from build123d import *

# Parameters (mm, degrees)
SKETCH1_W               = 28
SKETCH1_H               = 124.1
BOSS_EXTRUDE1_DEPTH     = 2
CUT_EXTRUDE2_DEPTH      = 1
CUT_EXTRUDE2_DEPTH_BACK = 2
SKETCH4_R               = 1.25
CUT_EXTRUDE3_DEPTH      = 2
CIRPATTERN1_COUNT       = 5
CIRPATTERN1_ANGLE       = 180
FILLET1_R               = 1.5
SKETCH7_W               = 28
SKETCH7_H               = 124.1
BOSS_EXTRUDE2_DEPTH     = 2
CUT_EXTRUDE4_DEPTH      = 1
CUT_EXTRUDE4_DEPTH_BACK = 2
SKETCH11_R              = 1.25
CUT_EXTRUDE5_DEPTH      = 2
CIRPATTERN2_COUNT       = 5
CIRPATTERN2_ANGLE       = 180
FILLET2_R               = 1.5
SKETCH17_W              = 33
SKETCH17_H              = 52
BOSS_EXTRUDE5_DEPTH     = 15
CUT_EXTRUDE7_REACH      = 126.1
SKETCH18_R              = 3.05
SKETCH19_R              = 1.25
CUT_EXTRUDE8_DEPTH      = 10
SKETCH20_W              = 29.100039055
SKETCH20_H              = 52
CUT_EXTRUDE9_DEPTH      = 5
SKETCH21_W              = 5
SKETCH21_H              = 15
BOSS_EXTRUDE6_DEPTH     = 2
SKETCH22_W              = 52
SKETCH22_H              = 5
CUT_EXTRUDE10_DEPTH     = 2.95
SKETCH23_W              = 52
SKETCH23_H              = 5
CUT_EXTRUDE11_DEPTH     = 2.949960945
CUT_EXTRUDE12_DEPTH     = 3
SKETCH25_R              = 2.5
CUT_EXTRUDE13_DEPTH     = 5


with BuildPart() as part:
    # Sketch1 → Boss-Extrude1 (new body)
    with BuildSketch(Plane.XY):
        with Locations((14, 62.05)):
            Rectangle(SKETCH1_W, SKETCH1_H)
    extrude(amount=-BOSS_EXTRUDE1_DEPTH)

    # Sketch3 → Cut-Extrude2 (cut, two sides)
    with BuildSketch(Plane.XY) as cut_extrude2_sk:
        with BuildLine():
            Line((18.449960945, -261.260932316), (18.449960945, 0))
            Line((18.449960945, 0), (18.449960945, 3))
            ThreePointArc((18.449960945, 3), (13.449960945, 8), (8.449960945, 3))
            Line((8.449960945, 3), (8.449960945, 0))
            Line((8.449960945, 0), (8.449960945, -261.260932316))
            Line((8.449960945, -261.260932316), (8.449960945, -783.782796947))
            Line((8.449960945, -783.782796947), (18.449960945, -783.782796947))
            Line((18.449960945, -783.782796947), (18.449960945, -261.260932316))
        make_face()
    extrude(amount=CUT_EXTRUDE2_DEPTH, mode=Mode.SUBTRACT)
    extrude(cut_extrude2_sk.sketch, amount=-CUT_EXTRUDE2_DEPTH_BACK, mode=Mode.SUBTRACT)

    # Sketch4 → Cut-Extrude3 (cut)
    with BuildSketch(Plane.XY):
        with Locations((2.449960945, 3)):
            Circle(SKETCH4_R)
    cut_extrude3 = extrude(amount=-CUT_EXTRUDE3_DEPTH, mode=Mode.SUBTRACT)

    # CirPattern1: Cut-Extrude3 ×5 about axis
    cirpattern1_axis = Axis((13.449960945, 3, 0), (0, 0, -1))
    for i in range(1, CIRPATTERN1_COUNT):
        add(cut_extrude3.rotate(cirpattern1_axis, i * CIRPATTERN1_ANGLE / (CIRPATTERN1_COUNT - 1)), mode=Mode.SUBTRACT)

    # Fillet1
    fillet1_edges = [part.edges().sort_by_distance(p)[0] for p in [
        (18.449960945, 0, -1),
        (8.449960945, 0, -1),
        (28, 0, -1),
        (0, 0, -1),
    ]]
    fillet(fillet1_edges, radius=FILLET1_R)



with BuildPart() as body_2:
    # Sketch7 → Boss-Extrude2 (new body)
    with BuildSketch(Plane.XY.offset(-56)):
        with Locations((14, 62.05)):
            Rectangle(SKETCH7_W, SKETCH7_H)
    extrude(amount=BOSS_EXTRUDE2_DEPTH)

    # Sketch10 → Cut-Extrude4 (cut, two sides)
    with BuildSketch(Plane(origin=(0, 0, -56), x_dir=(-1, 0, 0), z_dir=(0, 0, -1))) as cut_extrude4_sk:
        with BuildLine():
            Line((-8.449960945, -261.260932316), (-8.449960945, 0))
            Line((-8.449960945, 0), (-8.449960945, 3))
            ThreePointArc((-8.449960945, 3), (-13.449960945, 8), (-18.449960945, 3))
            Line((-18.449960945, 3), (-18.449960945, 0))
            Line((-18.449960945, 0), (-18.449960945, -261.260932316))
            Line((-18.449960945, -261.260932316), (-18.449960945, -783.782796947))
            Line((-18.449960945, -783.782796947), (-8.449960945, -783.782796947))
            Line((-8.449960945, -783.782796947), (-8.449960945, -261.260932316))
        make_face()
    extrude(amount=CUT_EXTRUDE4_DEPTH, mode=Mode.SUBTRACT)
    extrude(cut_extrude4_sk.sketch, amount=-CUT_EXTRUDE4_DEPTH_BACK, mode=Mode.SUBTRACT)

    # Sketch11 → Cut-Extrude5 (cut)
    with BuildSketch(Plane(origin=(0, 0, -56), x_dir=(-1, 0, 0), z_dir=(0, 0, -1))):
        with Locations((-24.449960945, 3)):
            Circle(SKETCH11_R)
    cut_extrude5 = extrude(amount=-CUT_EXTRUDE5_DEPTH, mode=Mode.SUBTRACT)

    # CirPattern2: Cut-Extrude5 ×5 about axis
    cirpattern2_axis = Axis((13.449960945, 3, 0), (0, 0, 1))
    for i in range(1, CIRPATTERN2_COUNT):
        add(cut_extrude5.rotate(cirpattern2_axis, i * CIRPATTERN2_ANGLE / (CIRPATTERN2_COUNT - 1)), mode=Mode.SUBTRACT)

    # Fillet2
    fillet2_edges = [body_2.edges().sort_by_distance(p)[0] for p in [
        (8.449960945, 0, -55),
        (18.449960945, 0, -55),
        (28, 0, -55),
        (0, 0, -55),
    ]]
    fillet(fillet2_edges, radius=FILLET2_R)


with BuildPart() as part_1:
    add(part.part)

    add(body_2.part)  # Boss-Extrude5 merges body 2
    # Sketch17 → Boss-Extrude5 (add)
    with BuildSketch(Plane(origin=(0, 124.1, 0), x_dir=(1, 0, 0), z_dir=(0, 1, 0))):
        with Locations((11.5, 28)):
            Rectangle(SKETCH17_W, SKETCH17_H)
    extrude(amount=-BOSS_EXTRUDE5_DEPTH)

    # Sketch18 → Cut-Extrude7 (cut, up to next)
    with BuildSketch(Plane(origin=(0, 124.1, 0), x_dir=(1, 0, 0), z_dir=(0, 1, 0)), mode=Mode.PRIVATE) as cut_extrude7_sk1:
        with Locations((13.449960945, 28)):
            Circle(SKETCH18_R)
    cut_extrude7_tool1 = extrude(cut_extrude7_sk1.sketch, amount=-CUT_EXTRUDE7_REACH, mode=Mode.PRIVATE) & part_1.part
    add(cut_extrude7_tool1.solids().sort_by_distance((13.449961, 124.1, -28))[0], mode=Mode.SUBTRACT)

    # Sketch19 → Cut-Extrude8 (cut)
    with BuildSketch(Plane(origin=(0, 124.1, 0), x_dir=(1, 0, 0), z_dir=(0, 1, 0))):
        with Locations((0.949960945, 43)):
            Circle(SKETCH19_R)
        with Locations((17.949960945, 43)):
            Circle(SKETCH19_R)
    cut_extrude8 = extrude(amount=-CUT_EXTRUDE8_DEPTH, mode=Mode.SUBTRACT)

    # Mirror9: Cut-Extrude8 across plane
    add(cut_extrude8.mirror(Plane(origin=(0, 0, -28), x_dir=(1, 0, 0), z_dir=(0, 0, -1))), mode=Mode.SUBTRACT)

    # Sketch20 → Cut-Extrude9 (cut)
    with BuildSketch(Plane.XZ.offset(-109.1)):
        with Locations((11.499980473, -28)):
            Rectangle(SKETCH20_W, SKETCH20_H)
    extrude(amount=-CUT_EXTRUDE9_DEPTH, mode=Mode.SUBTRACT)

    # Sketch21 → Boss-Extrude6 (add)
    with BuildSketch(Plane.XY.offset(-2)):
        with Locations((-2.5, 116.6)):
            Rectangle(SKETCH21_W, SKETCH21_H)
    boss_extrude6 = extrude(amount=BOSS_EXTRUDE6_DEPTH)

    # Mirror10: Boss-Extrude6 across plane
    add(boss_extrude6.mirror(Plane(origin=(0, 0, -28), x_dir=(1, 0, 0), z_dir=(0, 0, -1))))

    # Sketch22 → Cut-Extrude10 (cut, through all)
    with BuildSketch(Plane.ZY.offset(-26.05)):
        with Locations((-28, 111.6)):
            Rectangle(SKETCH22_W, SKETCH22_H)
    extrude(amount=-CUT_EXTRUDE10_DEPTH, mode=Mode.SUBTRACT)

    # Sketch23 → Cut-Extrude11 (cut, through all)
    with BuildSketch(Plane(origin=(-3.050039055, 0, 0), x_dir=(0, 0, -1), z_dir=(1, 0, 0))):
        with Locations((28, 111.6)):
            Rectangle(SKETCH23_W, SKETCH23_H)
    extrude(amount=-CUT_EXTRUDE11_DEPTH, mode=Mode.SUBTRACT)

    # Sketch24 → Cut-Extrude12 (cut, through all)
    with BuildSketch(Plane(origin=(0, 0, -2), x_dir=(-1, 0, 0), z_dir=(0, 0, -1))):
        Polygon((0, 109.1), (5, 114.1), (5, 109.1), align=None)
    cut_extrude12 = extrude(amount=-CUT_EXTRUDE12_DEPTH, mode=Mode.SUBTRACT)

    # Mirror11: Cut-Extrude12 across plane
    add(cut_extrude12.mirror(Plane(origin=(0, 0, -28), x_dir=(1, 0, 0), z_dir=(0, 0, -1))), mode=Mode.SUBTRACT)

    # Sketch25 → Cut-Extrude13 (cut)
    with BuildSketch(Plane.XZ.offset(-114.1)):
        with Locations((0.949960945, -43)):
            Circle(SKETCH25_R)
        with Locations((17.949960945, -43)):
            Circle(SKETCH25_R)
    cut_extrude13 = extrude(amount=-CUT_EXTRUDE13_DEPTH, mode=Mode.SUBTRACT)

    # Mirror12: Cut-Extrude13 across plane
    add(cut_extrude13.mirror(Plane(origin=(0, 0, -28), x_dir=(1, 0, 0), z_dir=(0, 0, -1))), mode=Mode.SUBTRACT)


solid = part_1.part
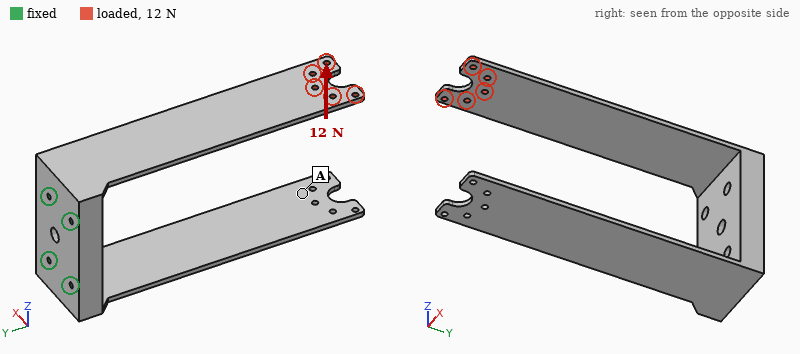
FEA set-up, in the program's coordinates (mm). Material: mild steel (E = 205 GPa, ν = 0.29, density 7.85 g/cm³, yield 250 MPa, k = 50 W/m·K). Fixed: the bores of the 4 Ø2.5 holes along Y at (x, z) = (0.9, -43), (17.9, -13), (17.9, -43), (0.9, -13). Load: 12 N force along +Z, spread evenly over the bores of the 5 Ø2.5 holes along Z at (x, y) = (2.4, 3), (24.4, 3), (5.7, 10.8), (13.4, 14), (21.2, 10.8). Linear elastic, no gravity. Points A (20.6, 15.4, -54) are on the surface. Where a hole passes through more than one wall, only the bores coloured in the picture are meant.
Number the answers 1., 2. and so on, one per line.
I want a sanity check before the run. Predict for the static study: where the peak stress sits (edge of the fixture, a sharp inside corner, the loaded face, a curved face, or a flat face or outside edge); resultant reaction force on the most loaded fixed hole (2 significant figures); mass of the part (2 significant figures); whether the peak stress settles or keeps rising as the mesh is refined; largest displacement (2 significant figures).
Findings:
1. a sharp inside corner
2. 38 N
3. 240 g
4. keeps rising
5. 1.4 mm
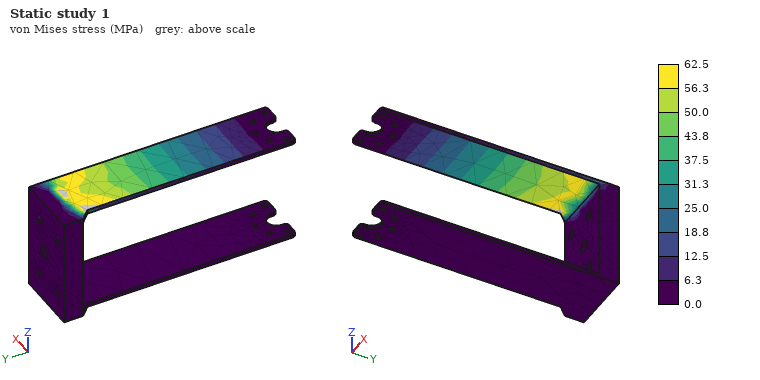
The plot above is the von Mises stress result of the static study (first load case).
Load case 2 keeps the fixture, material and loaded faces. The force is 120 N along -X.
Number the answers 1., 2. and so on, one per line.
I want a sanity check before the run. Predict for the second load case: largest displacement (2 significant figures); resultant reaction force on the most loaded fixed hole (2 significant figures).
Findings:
1. 0.11 mm
2. 730 N
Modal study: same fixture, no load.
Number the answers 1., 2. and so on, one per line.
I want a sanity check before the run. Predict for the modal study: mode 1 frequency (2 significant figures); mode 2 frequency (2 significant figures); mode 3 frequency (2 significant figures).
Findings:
1. 130 Hz
2. 130 Hz
3. 830 Hz
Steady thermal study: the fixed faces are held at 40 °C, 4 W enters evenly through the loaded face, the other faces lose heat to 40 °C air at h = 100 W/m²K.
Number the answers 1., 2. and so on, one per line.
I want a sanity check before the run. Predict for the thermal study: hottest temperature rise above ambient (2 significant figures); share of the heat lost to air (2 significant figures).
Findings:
1. 27 K
2. 99 %
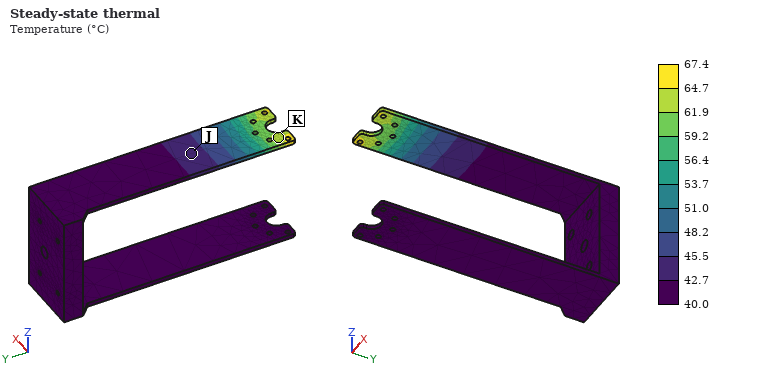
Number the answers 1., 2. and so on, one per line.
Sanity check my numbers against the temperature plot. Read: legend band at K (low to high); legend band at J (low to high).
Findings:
1. 61.9 to 64.7 °C
2. 42.7 to 45.5 °C
